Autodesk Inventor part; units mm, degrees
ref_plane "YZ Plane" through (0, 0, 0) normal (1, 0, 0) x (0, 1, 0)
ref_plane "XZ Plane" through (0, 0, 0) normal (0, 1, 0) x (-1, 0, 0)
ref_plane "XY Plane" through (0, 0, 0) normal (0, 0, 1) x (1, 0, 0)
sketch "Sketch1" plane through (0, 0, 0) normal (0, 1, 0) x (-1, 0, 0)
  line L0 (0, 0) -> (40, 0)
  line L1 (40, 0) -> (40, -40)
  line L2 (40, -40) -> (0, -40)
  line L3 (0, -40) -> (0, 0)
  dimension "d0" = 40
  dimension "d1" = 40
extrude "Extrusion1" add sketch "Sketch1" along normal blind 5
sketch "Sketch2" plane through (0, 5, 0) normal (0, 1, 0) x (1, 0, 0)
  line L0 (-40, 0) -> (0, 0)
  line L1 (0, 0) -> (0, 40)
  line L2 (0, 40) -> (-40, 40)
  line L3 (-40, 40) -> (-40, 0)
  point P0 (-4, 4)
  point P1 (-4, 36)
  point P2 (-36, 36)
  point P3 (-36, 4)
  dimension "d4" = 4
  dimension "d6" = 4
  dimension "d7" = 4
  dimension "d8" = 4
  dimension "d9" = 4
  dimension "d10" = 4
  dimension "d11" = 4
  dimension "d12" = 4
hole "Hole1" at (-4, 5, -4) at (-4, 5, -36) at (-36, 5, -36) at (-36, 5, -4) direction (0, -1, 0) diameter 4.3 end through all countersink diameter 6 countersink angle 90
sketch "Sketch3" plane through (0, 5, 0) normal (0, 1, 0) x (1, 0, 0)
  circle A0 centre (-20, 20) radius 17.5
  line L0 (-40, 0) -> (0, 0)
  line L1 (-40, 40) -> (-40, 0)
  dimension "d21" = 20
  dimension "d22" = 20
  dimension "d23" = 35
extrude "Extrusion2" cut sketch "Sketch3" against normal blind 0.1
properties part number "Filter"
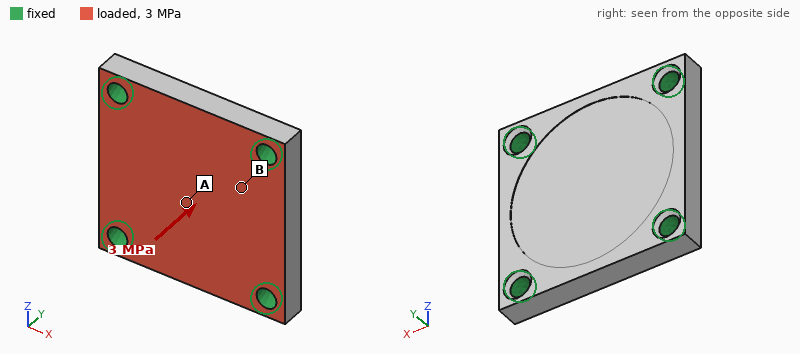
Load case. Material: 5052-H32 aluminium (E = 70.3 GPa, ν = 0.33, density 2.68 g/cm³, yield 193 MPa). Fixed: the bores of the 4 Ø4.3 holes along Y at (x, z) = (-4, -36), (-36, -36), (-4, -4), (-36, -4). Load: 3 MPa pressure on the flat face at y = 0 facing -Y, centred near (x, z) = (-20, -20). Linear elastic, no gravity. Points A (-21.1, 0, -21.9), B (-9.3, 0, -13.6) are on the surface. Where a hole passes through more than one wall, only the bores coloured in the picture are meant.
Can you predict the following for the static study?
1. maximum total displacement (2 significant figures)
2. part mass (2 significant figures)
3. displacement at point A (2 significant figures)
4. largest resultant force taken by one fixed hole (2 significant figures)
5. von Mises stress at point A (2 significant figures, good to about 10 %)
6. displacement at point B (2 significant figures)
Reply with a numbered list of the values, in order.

1. 31 µm
2. 20 g
3. 31 µm
4. 1.2 kN
5. 36 MPa
6. 20 µm
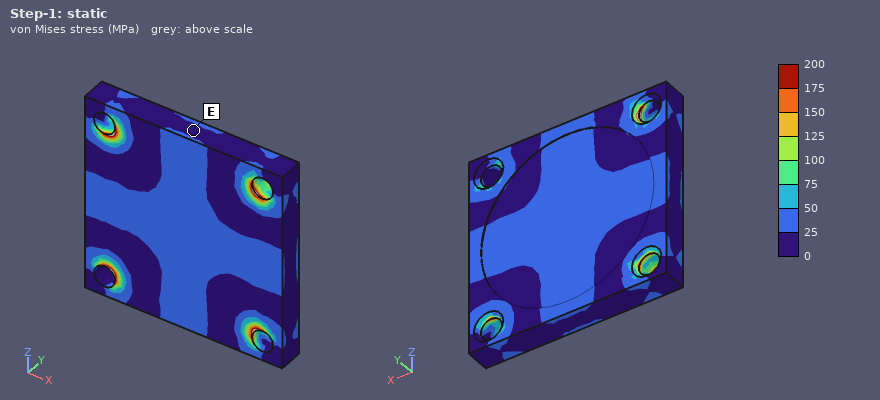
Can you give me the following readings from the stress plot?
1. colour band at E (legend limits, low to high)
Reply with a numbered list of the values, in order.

1. 0 to 25 MPa
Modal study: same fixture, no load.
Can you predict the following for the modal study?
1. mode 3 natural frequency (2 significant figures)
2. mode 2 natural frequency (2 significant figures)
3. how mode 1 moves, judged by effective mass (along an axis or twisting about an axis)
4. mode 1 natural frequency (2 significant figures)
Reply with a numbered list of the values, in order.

1. 26 kHz
2. 26 kHz
3. along Y
4. 16 kHz
